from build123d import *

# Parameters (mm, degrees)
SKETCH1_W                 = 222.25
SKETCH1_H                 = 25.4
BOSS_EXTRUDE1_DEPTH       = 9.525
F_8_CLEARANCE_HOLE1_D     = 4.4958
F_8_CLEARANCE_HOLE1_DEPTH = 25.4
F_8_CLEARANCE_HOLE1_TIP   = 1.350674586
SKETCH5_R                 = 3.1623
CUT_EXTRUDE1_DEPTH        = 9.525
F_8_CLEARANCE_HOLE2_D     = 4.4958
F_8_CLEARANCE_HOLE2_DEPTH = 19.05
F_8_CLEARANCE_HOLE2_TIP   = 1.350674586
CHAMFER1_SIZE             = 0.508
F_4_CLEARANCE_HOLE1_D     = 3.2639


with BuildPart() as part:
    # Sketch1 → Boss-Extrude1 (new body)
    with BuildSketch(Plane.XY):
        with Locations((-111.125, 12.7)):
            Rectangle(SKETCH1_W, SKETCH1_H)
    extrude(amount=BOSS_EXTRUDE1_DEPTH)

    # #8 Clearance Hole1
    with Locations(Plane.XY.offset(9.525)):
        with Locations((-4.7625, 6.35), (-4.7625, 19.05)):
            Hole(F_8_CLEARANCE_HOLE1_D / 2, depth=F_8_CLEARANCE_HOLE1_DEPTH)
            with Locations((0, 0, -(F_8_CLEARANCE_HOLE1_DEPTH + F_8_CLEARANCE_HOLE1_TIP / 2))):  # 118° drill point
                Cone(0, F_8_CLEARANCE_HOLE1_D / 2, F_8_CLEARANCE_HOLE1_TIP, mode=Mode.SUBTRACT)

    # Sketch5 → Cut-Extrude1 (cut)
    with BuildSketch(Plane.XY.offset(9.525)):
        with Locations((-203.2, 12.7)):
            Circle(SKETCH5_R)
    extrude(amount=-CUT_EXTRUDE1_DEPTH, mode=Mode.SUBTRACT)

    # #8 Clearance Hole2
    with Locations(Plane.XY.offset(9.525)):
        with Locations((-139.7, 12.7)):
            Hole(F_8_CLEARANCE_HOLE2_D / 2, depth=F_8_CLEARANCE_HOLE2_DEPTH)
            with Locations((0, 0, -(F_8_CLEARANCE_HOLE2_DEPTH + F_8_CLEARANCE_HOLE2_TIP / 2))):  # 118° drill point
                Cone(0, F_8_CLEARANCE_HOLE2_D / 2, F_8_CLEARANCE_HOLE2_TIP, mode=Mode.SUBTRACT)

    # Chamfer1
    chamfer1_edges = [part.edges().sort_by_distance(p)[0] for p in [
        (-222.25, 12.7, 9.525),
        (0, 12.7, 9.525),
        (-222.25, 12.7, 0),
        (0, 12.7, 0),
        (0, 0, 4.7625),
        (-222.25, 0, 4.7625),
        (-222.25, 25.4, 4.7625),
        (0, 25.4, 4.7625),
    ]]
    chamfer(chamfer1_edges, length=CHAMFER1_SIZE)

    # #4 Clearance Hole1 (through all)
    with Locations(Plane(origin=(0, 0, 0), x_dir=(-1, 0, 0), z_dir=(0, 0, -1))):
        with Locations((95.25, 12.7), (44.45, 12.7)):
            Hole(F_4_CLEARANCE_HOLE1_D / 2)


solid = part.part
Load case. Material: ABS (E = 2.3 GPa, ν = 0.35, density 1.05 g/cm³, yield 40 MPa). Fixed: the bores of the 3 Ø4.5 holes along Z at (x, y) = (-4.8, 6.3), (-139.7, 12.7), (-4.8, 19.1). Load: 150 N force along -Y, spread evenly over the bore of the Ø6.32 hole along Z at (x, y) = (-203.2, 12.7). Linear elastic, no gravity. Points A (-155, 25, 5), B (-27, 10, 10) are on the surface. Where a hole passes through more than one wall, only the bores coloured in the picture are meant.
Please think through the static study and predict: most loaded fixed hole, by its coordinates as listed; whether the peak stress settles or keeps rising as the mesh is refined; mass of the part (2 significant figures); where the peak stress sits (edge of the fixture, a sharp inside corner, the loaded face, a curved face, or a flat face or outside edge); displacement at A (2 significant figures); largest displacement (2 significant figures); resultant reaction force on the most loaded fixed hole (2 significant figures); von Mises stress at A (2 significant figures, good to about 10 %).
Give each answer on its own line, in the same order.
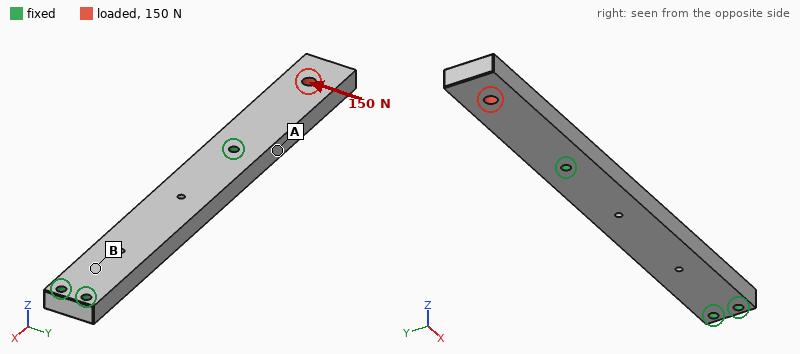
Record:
(-139.7, 12.7)
keeps rising
55 g
edge of the fixture
0.22 mm
1.3 mm
210 N
7.1 MPa
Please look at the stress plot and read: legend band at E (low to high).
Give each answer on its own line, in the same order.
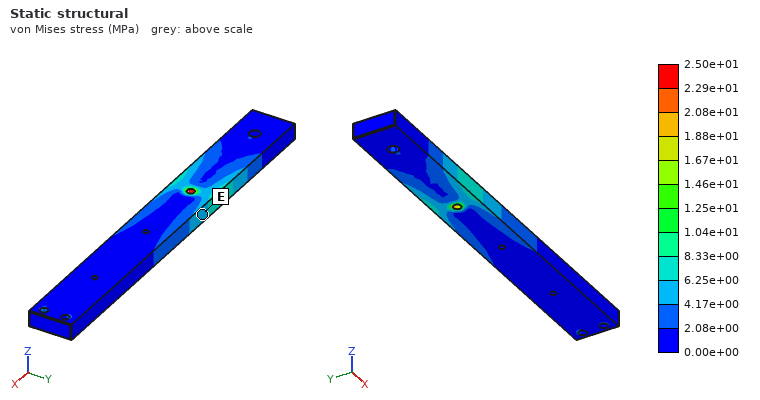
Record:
4.17e+00 to 6.25e+00 MPa
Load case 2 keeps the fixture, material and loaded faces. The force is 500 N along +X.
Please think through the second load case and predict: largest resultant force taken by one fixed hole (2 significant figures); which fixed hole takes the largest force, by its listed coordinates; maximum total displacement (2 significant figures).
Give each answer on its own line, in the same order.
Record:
480 N
(-139.7, 12.7)
72 µm
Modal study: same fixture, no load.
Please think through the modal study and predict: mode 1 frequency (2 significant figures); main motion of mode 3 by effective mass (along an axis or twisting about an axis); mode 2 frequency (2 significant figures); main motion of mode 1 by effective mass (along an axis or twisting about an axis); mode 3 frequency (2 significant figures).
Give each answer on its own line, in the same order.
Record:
320 Hz
along Z
590 Hz
along Z
770 Hz
